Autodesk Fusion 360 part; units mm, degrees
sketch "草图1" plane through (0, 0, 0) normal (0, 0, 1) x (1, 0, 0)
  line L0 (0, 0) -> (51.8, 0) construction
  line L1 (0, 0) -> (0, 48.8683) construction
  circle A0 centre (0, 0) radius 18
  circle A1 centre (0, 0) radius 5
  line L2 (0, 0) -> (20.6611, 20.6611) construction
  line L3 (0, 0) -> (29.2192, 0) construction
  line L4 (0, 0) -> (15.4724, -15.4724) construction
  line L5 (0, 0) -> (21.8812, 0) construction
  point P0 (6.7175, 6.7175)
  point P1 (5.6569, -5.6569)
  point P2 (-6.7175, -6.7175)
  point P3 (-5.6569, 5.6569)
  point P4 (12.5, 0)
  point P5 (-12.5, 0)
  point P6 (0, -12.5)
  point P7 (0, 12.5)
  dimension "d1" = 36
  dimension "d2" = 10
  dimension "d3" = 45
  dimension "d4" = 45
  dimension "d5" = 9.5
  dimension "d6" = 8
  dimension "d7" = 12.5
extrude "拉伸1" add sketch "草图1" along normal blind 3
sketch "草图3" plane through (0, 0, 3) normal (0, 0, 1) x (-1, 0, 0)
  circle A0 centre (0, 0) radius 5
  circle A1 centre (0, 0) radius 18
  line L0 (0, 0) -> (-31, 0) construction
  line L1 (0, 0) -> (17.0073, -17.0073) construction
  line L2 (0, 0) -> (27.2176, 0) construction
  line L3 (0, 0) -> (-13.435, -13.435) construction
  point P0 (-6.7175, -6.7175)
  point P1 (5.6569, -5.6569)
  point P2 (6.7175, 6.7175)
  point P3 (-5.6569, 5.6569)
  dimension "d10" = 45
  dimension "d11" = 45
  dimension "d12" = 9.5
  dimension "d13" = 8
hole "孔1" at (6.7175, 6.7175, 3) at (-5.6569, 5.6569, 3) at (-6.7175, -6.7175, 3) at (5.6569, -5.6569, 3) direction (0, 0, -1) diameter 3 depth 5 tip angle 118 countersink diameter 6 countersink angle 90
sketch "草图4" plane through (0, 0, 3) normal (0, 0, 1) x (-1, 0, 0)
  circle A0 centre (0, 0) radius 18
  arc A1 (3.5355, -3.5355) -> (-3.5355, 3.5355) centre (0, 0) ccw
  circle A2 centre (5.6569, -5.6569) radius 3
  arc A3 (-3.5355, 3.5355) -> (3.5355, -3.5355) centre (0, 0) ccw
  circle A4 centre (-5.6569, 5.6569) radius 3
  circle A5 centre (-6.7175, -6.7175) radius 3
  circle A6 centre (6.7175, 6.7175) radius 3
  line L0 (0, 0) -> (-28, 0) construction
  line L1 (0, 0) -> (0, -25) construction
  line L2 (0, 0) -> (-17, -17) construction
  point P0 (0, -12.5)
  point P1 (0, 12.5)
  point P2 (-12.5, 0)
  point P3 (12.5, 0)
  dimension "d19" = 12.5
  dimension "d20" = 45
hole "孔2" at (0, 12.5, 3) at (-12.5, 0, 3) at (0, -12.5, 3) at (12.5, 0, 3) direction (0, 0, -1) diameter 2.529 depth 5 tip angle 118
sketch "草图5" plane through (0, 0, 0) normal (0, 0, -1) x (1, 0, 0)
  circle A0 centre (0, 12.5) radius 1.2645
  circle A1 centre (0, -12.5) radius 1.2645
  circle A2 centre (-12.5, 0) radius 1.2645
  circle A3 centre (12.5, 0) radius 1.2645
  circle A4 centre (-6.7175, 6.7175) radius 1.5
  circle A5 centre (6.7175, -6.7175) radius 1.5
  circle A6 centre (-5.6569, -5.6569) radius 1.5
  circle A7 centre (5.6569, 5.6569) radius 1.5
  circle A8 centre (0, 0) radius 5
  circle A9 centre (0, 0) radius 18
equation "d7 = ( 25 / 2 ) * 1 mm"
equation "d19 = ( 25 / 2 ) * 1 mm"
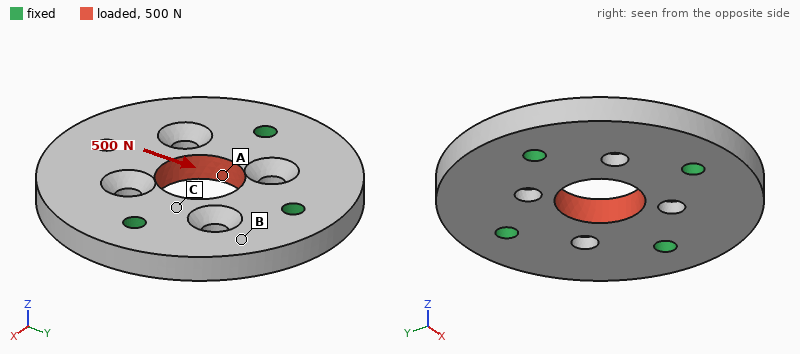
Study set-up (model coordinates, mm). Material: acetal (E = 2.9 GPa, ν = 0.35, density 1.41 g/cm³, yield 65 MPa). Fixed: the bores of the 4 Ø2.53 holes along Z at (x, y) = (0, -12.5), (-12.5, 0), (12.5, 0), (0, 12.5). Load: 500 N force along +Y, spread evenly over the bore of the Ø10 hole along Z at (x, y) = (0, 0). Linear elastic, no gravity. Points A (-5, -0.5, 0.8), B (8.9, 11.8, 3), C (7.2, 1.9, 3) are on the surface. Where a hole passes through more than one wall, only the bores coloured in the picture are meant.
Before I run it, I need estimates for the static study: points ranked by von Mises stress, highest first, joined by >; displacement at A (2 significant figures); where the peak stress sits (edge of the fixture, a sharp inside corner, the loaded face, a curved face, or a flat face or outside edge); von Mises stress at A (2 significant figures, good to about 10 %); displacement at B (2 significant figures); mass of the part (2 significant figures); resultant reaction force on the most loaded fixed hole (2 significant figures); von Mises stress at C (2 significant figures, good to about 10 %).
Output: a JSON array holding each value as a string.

["A > C > B", "27 µm", "a curved face", "9.4 MPa", "8.5 µm", "3.7 g", "150 N", "4.2 MPa"]
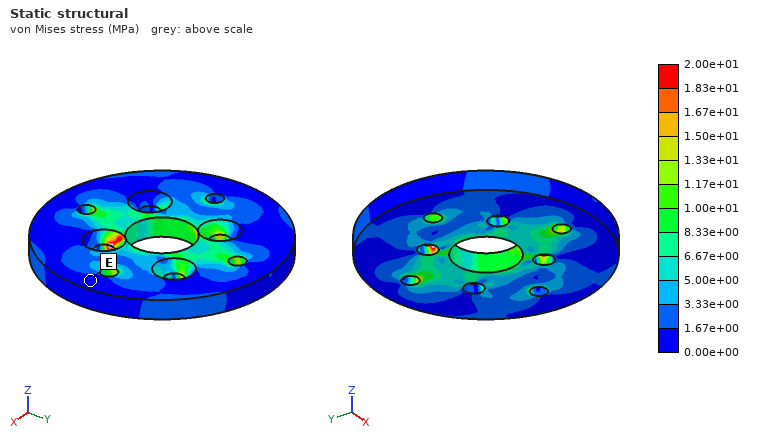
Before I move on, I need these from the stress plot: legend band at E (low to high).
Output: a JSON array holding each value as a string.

["0.00e+00 to 1.67e+00 MPa"]
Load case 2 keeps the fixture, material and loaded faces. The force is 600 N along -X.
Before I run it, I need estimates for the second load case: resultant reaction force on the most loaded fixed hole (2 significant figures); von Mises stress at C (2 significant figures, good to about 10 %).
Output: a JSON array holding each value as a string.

["190 N", "7.9 MPa"]
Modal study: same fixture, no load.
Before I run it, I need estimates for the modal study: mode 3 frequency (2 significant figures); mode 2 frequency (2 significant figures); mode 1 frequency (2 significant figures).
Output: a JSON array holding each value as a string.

["7600 Hz", "7600 Hz", "7000 Hz"]
